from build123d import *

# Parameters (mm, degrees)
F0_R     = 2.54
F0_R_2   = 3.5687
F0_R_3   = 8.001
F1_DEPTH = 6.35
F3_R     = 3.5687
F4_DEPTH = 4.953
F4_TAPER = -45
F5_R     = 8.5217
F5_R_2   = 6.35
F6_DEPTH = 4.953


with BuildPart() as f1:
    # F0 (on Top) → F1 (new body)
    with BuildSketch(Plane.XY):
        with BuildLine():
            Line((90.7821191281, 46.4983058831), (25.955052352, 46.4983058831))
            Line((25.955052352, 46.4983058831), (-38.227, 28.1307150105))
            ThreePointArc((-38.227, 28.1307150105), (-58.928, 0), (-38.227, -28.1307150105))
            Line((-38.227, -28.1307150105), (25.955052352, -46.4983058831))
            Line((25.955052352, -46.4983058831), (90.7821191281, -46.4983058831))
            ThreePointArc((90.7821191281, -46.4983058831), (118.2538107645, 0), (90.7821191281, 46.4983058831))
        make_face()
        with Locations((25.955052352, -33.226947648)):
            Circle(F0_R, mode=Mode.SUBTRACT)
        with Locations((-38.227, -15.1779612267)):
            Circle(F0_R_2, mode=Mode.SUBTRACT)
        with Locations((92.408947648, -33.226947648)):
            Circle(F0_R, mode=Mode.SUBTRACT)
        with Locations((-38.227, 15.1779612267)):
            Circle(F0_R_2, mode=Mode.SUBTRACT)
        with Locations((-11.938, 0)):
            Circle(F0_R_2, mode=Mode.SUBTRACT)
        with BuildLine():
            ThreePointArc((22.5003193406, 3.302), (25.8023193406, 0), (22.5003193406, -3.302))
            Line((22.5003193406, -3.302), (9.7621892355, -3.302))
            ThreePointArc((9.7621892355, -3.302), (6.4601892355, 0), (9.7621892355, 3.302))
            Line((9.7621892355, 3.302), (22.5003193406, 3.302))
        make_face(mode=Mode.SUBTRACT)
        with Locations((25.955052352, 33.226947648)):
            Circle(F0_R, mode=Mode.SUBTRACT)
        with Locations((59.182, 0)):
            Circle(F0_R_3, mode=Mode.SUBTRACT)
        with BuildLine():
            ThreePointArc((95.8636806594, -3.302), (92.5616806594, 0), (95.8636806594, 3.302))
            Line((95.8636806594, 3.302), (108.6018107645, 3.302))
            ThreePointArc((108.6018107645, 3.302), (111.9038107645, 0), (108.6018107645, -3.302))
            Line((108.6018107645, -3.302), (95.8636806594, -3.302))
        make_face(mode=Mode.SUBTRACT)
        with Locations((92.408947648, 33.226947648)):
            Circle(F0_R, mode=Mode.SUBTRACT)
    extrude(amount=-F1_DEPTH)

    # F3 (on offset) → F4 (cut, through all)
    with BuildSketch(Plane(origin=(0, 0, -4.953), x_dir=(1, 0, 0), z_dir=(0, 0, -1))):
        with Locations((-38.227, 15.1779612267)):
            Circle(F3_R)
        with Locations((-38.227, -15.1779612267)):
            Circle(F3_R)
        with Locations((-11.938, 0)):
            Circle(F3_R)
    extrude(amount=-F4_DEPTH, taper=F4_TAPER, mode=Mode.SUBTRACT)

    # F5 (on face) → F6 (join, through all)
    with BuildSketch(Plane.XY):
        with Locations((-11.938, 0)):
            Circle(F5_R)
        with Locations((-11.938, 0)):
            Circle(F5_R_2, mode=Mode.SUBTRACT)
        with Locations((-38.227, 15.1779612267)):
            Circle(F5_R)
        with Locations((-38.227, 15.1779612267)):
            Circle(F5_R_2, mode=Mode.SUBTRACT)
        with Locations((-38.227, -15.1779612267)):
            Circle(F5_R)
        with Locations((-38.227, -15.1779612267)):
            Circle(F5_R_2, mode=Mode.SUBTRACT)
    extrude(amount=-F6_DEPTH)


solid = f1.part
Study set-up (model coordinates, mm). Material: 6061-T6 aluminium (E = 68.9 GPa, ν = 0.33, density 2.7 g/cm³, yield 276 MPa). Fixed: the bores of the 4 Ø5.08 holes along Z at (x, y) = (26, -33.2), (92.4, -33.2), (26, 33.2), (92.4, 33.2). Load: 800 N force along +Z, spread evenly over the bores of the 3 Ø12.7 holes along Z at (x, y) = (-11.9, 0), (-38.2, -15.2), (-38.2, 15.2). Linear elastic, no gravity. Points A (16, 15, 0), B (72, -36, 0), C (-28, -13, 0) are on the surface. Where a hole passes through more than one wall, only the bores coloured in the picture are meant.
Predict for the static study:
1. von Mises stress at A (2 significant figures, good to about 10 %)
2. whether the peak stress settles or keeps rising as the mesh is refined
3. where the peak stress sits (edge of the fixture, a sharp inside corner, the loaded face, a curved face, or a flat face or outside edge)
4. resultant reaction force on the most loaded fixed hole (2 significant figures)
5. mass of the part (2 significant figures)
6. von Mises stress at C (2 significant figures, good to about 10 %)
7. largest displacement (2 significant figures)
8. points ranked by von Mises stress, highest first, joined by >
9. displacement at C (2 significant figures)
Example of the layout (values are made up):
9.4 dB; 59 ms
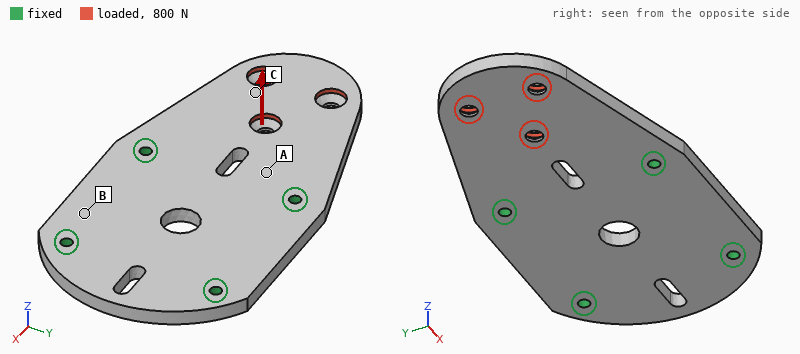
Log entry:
56 MPa; keeps rising; edge of the fixture; 510 N; 220 g; 22 MPa; 0.89 mm; A > C > B; 0.47 mm
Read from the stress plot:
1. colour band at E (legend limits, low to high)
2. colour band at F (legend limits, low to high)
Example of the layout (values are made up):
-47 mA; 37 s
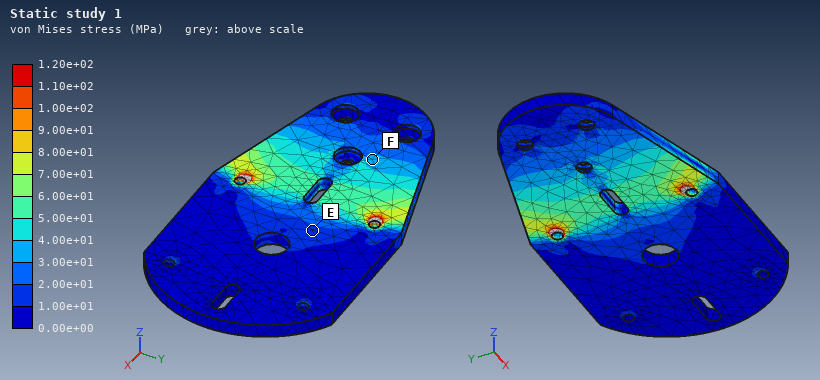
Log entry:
1.00e+01 to 2.00e+01 MPa; 3.00e+01 to 4.00e+01 MPa
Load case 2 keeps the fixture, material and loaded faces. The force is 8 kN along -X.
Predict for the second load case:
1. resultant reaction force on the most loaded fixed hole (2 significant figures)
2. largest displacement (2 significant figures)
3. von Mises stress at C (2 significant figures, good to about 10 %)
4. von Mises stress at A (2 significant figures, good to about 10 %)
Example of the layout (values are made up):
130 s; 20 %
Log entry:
3.4 kN; 0.55 mm; 43 MPa; 40 MPa
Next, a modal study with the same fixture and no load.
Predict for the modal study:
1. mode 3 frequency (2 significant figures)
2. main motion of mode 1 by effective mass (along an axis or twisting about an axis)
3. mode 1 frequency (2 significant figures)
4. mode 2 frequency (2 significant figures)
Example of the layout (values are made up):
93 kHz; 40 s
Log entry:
4300 Hz; along Z; 880 Hz; 3000 Hz
